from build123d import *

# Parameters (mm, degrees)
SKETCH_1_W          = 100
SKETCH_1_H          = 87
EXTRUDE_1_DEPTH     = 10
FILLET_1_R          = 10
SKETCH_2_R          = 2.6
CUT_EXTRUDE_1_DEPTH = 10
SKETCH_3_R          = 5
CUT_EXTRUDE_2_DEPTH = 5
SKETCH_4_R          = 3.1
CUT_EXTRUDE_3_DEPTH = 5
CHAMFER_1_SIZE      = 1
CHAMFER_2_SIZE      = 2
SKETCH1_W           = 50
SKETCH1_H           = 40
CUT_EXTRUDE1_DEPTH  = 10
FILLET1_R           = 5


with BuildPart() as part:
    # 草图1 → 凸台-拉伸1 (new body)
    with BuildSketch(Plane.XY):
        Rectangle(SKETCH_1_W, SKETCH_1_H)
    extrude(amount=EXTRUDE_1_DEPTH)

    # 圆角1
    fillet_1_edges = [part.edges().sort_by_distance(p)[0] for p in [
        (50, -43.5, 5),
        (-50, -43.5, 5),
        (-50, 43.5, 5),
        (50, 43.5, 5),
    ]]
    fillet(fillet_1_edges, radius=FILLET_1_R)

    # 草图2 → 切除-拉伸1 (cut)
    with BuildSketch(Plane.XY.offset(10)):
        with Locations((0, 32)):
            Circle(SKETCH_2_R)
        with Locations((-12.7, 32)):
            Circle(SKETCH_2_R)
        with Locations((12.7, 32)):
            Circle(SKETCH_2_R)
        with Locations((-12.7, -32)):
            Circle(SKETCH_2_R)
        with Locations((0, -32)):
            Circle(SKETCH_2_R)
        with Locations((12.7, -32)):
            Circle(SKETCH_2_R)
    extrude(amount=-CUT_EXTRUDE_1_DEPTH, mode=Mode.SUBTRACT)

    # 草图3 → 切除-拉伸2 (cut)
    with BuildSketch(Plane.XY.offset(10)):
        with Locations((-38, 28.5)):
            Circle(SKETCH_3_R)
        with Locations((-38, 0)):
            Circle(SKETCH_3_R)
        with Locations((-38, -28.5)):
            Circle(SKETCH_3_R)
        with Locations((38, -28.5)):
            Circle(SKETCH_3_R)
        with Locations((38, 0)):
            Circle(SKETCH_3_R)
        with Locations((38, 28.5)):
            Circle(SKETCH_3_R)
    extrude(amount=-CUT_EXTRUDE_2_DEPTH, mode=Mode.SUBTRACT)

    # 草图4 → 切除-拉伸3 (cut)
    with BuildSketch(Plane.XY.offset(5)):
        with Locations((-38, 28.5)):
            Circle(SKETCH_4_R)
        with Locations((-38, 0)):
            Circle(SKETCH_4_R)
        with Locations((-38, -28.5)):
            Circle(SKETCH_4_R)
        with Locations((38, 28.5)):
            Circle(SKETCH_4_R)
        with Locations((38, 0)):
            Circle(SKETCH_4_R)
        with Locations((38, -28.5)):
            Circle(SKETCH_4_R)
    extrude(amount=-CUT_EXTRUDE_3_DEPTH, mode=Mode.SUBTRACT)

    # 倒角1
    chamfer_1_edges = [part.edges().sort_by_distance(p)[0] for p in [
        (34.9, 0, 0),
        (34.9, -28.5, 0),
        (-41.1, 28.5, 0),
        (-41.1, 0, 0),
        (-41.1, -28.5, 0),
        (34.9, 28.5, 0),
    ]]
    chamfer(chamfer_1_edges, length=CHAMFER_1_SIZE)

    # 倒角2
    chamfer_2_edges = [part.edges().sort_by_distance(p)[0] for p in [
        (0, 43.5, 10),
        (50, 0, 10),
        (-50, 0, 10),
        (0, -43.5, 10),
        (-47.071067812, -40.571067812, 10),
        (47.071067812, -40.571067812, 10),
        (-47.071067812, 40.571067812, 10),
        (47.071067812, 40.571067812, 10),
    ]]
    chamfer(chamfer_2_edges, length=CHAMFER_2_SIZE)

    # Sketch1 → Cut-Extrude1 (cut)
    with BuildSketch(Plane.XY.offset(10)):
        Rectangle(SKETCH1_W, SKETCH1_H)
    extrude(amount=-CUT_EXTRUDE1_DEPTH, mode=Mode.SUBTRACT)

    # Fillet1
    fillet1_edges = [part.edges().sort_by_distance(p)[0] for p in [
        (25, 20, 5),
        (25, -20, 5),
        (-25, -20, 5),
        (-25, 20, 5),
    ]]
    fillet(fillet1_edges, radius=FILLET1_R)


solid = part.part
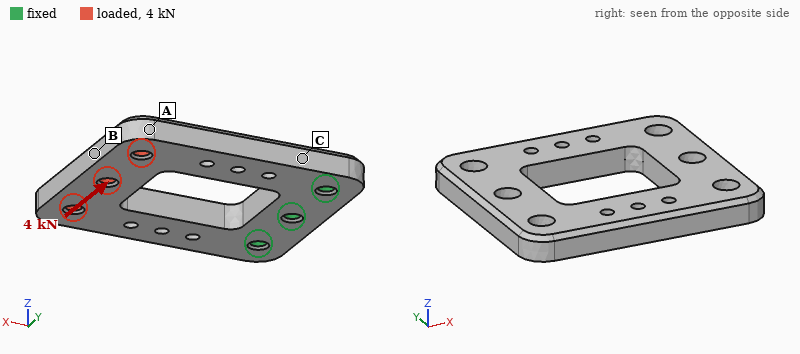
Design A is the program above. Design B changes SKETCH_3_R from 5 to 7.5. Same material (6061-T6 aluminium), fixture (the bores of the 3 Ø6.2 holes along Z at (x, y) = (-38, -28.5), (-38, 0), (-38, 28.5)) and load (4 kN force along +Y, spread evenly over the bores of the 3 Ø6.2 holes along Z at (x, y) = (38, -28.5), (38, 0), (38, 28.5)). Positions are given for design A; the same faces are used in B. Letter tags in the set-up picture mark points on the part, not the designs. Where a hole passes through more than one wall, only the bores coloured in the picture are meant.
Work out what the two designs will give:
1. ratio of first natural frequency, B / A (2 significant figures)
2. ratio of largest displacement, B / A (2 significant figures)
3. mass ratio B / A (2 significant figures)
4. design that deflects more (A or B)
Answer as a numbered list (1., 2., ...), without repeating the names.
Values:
1. 0.99
2. 1.1
3. 0.95
4. B
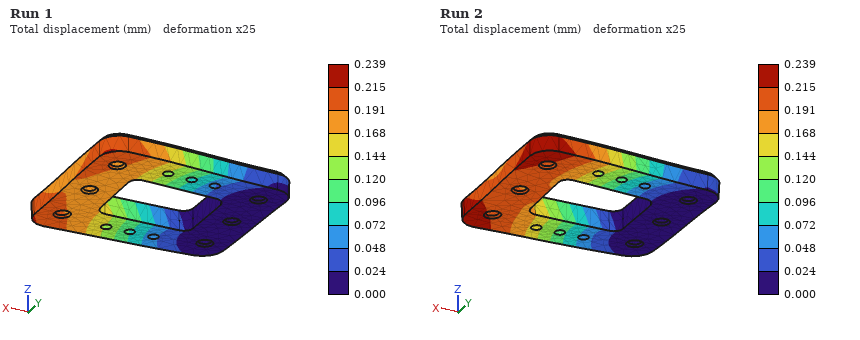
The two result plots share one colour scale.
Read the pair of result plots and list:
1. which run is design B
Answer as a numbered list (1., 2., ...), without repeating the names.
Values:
1. Run 2
